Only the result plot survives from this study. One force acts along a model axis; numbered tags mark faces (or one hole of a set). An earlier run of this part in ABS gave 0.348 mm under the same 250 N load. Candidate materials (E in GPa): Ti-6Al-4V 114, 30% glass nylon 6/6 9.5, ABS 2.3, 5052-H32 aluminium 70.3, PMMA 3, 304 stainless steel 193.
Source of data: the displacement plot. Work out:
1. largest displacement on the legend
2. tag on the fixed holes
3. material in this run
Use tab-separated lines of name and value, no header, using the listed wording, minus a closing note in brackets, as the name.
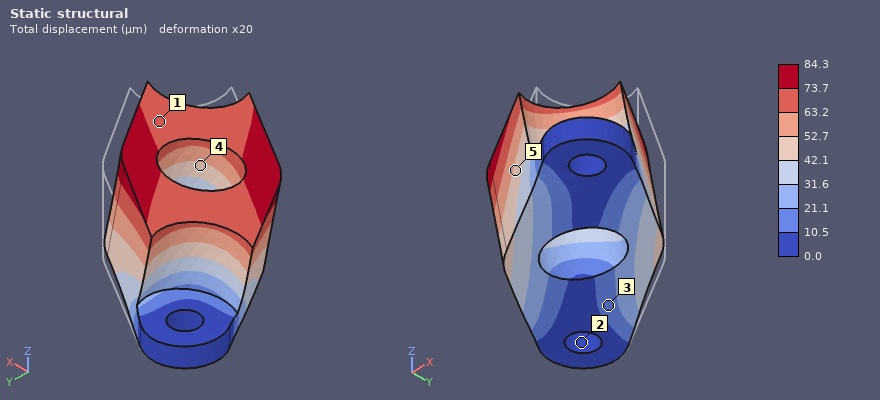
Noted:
largest displacement on the legend	84.3 µm
tag on the fixed holes	2
material in this run	30% glass nylon 6/6
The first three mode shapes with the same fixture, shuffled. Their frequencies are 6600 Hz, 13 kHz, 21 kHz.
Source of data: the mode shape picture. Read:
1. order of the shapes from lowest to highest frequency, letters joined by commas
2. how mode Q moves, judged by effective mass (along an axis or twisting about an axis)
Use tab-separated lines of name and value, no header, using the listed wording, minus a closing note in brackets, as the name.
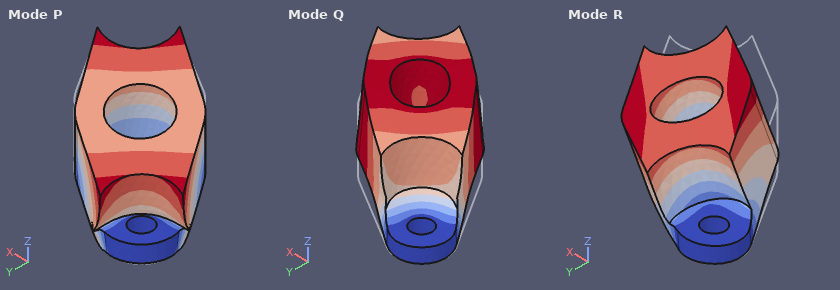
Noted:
order of the shapes from lowest to highest frequency, letters joined by commas	R, Q, P
how mode Q moves, judged by effective mass	along Z
